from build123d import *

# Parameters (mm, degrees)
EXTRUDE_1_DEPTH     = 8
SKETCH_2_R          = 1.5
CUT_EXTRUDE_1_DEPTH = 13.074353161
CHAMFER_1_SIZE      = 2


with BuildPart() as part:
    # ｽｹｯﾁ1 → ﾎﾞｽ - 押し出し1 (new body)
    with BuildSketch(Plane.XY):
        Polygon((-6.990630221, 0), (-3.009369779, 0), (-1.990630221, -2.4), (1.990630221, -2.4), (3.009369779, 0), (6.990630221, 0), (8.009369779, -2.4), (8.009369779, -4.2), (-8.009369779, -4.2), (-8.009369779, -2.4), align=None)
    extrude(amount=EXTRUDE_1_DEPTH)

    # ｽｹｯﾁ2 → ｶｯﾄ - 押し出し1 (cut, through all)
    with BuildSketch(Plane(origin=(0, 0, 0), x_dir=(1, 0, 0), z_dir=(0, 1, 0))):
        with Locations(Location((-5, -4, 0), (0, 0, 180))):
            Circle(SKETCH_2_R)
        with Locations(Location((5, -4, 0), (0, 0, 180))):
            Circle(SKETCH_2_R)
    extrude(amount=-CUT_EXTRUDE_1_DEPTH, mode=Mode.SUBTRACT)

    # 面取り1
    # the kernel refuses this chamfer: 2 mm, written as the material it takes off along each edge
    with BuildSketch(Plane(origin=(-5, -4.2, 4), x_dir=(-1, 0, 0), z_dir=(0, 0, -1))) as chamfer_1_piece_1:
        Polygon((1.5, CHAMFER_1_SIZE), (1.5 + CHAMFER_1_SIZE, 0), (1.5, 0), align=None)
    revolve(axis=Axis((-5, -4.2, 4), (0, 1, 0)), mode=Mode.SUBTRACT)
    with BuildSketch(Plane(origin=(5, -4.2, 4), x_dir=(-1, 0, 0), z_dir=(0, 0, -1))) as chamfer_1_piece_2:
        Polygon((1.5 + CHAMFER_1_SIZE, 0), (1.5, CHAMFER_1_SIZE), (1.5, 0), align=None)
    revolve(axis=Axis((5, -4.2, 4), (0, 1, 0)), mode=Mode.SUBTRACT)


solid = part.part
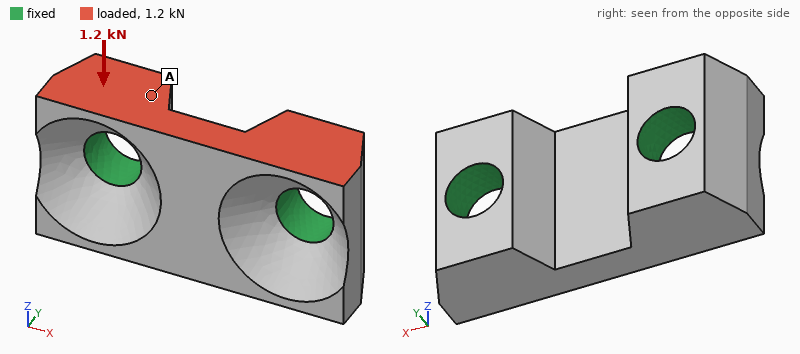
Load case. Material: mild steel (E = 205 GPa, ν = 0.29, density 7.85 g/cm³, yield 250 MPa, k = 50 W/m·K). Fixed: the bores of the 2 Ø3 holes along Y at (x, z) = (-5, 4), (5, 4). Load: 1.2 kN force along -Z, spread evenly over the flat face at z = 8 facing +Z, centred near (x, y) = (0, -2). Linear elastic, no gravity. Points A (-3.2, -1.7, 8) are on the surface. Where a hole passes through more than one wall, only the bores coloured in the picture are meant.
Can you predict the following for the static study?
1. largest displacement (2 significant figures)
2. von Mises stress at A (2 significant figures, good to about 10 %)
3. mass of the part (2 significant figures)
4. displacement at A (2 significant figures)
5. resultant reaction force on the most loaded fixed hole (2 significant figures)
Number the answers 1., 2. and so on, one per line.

1. 2.7 µm
2. 33 MPa
3. 2.4 g
4. 1.5 µm
5. 600 N
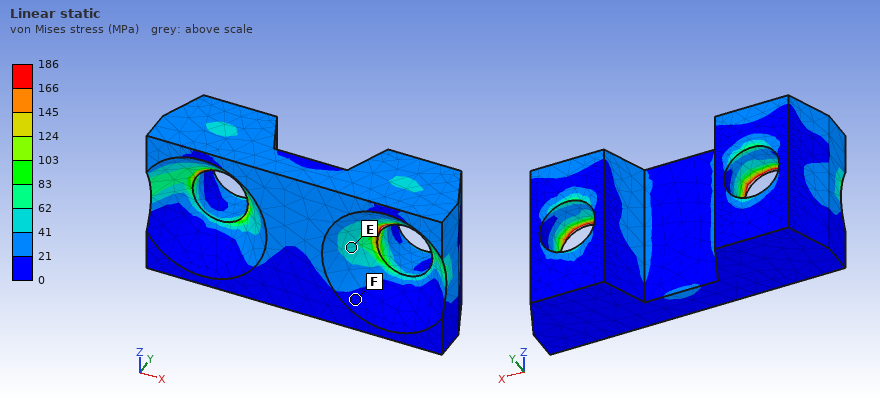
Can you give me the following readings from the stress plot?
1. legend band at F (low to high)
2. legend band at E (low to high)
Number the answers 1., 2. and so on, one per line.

1. 0 to 21 MPa
2. 41 to 62 MPa
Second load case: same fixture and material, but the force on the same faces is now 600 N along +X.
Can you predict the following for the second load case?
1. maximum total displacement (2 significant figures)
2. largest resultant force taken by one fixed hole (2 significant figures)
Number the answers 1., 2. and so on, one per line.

1. 1.8 µm
2. 320 N
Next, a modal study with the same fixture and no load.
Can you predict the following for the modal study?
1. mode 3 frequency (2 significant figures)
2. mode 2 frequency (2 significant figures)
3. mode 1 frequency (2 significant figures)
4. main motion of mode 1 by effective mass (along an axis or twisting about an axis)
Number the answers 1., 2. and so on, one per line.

1. 120 kHz
2. 110 kHz
3. 85 kHz
4. along Z
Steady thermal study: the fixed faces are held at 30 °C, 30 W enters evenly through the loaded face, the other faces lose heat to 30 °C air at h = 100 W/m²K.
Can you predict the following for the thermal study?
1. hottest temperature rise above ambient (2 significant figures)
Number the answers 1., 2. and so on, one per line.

1. 58 K
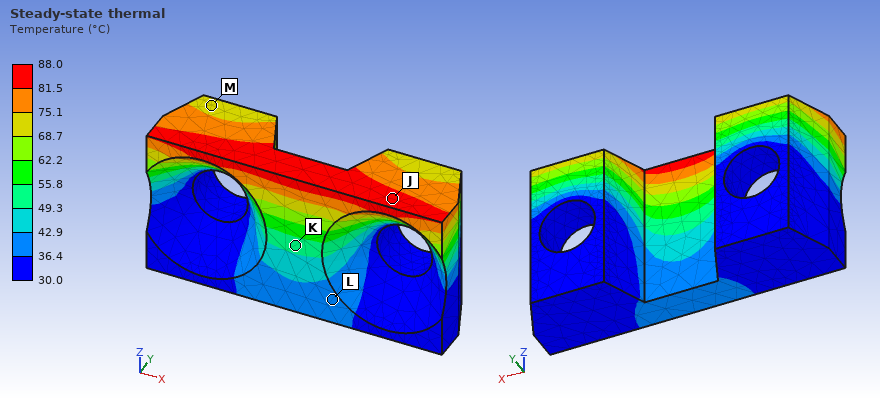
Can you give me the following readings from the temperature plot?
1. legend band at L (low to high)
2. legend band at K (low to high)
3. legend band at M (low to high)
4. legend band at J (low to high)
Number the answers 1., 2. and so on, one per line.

1. 36.4 to 42.9 °C
2. 49.3 to 55.8 °C
3. 68.7 to 75.1 °C
4. 81.5 to 88.0 °C
